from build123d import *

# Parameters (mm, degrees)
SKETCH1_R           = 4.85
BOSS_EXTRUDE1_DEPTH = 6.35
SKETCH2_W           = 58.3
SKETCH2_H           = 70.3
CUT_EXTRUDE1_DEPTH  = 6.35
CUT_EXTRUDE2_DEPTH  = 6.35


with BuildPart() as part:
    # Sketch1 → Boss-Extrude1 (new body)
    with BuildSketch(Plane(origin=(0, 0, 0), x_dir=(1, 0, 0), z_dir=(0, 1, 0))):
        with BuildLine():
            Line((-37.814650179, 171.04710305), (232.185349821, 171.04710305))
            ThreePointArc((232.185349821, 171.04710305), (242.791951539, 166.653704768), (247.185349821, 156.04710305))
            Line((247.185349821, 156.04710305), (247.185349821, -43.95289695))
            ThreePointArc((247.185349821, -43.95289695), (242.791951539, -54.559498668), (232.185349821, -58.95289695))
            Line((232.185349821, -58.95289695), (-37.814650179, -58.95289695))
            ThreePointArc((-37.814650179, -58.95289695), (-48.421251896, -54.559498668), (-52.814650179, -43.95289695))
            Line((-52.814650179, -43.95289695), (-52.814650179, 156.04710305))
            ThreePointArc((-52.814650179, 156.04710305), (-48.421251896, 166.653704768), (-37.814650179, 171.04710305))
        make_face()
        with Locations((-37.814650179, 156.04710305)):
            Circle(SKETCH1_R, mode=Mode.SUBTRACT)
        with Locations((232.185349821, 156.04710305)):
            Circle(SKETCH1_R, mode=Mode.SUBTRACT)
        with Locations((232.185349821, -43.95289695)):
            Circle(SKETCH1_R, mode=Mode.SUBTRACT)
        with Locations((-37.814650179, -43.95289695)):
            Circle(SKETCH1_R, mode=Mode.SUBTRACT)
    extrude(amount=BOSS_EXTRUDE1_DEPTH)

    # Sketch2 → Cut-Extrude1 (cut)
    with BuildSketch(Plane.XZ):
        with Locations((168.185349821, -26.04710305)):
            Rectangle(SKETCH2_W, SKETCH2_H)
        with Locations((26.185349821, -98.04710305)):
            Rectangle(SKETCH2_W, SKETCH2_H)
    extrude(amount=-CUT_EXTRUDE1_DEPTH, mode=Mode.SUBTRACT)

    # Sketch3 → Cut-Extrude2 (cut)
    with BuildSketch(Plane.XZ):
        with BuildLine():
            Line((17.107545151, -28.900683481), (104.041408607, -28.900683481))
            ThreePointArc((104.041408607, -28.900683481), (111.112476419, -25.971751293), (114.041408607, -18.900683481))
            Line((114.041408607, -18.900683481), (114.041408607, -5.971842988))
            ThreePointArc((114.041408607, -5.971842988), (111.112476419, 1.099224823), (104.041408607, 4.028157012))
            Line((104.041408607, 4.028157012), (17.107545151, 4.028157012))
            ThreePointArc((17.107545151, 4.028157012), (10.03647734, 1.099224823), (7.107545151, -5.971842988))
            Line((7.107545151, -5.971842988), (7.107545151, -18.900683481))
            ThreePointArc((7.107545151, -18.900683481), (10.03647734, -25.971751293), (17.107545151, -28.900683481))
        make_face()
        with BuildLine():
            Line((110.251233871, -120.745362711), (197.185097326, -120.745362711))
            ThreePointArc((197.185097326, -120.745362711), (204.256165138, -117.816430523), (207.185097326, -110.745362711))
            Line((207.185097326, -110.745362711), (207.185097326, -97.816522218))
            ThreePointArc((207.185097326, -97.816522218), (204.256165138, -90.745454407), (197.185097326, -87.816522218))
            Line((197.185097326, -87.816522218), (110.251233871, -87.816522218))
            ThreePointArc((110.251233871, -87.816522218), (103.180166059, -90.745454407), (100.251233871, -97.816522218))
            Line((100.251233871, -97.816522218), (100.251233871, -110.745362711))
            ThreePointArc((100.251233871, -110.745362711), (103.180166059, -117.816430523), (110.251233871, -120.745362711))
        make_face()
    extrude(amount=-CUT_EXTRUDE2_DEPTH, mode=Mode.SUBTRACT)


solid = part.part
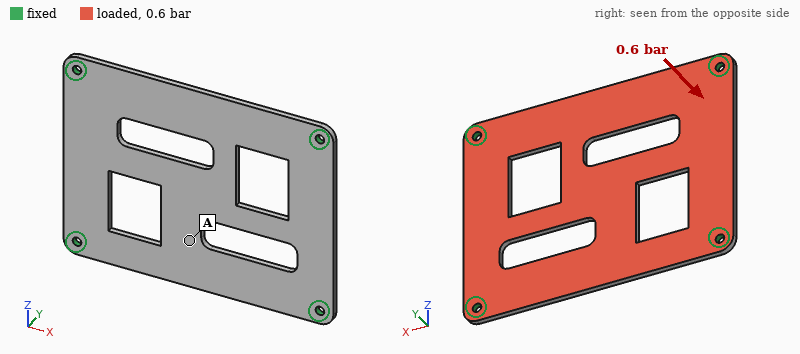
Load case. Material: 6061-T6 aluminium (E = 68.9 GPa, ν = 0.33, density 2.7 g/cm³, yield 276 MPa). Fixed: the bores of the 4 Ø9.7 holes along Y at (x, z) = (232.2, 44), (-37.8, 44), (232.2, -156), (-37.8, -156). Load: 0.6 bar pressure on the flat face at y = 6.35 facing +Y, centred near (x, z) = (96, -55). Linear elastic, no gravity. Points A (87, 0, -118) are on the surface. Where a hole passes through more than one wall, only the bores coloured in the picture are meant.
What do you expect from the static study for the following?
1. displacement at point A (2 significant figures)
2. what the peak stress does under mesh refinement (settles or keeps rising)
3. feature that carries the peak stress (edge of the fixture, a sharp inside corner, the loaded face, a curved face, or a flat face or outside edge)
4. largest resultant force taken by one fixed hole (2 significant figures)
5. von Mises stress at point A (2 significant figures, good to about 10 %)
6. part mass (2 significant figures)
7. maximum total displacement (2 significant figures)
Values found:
0.87 mm
keeps rising
edge of the fixture
840 N
19 MPa
920 g
1.0 mm
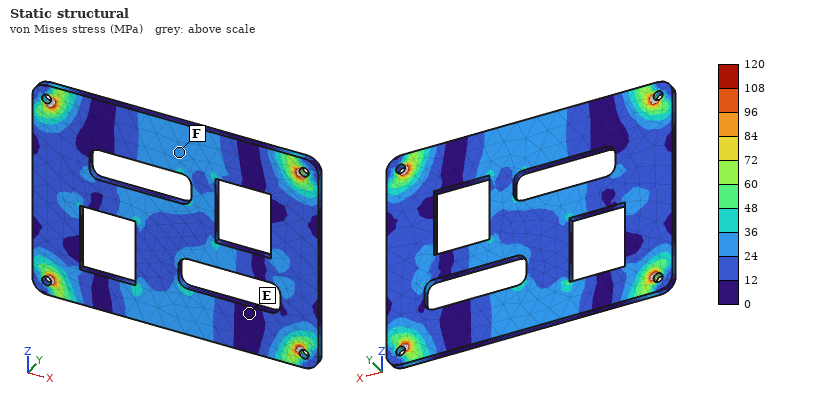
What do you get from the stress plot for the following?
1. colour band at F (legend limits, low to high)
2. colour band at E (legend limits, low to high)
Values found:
24 to 36 MPa
0 to 12 MPa
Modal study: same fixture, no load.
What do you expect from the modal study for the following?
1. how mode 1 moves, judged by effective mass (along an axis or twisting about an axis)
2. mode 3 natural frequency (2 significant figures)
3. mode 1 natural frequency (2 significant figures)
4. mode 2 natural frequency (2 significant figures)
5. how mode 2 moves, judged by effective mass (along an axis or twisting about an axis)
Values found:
along Y
710 Hz
360 Hz
520 Hz
twisting about X
